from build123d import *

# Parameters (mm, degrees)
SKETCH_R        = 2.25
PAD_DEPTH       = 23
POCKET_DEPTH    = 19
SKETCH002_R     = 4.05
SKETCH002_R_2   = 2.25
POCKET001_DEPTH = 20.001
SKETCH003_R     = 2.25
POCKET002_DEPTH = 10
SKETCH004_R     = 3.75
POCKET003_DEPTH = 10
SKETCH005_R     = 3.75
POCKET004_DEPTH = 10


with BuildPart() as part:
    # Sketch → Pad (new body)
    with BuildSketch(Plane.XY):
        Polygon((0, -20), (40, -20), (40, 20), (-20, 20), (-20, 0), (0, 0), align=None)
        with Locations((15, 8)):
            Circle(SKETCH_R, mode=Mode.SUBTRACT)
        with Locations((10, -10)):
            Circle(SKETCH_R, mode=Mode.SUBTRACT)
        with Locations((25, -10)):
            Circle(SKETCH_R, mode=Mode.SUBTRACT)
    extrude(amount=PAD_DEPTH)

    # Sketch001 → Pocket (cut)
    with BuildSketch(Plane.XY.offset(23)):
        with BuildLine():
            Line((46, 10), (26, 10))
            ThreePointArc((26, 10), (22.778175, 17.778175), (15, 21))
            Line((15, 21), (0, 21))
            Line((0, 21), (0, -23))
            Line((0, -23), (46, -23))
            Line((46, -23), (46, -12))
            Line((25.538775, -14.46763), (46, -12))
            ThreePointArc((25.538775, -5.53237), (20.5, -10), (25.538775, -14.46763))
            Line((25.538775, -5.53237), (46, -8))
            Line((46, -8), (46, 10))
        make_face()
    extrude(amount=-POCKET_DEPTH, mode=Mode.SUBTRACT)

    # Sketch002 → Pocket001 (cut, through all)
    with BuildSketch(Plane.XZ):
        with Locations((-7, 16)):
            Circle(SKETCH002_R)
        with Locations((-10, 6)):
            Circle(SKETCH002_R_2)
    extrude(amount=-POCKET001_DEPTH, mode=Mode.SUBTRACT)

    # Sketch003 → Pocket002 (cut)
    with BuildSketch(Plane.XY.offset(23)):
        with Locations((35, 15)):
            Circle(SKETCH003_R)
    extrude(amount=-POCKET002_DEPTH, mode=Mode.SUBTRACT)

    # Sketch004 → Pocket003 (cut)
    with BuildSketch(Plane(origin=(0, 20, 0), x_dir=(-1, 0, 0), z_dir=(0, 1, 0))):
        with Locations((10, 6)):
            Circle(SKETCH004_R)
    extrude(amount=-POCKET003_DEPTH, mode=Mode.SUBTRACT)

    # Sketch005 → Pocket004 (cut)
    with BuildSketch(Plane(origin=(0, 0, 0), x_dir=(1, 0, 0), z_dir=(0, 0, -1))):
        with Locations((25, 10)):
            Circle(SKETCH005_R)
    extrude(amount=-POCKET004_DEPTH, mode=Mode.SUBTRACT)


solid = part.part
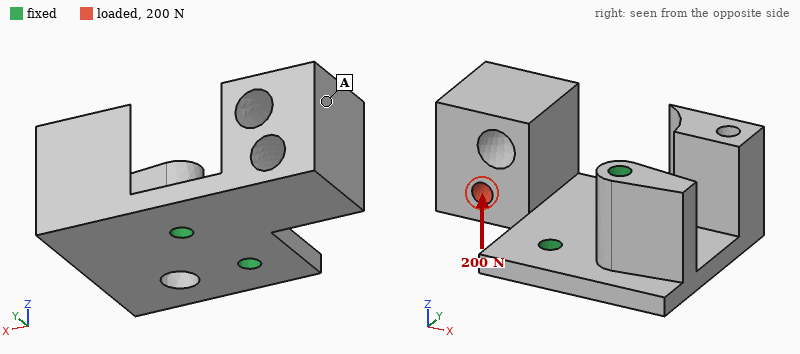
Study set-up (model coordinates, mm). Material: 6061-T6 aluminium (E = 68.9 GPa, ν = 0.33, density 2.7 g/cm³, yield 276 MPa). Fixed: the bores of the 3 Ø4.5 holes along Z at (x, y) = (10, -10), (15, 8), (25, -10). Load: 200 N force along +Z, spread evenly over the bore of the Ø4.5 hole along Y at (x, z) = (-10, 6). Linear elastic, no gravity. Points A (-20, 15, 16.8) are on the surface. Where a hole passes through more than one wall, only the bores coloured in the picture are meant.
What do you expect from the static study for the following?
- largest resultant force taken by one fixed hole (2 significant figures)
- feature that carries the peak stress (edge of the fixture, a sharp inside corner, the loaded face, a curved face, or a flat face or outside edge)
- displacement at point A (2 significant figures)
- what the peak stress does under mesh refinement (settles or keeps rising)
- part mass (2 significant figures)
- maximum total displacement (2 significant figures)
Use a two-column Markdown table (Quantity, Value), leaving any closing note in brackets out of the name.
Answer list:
| Quantity | Value |
|---|---|
| largest resultant force taken by one fixed hole | 120 N |
| feature that carries the peak stress | edge of the fixture |
| displacement at point A | 0.15 mm |
| what the peak stress does under mesh refinement | keeps rising |
| part mass | 51 g |
| maximum total displacement | 0.17 mm |
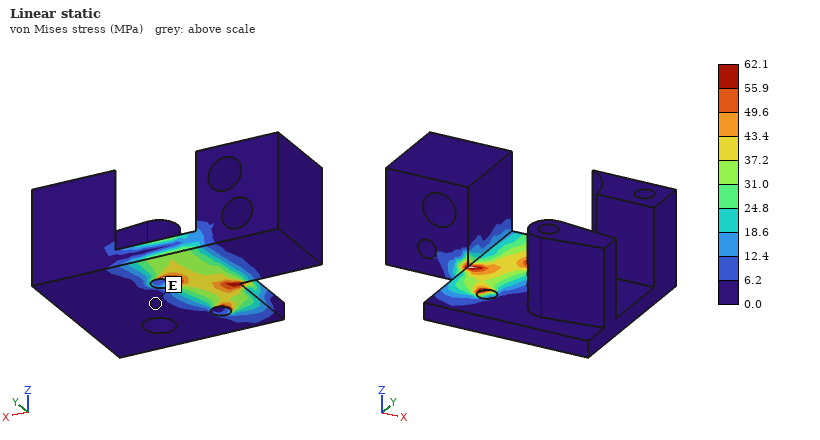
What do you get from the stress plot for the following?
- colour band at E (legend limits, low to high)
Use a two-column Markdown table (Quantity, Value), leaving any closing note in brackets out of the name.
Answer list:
| Quantity | Value |
|---|---|
| colour band at E | 0.0 to 6.2 MPa |
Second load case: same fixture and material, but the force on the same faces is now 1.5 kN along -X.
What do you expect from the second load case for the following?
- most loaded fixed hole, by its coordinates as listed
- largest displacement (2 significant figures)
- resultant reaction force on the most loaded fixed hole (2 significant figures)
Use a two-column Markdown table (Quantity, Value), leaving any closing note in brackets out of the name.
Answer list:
| Quantity | Value |
|---|---|
| most loaded fixed hole, by its coordinates as listed | (15, 8) |
| largest displacement | 0.33 mm |
| resultant reaction force on the most loaded fixed hole | 1.2 kN |
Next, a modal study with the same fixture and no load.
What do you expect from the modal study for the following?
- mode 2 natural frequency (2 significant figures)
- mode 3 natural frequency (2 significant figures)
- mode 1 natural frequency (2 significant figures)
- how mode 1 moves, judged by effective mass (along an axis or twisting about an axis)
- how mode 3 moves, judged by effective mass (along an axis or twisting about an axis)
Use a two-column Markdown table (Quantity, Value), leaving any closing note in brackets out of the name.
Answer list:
| Quantity | Value |
|---|---|
| mode 2 natural frequency | 3000 Hz |
| mode 3 natural frequency | 3300 Hz |
| mode 1 natural frequency | 1300 Hz |
| how mode 1 moves, judged by effective mass | along Z |
| how mode 3 moves, judged by effective mass | along Y |
